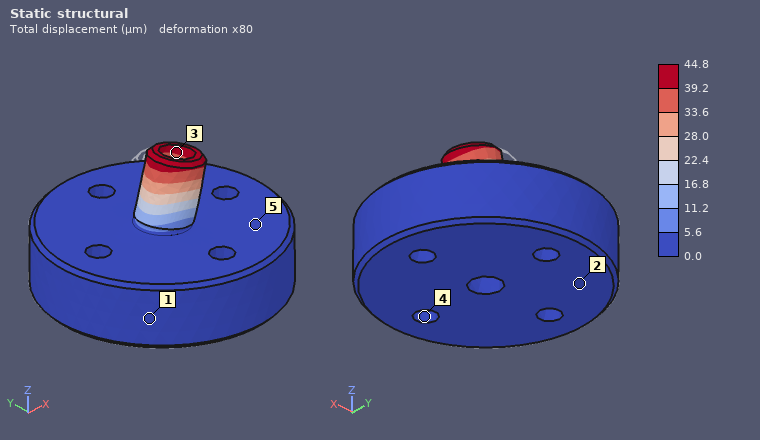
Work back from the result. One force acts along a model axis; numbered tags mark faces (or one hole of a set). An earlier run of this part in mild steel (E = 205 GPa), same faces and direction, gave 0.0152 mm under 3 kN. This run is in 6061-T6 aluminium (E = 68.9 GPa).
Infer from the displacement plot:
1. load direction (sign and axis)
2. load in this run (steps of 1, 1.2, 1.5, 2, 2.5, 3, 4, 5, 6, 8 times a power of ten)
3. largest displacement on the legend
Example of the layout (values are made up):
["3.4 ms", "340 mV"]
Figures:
["+X", "3 kN", "44.8 µm"]
